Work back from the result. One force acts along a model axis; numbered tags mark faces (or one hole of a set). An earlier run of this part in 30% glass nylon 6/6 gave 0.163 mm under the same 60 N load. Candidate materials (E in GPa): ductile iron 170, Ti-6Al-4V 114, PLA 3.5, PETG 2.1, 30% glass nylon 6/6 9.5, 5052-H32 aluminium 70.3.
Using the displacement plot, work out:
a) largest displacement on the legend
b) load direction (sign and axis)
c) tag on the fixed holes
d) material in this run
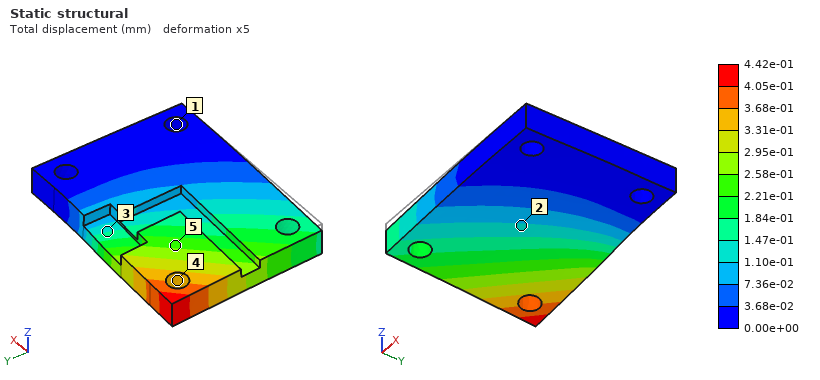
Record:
4.42e-01 mm
-Z
1
PLA
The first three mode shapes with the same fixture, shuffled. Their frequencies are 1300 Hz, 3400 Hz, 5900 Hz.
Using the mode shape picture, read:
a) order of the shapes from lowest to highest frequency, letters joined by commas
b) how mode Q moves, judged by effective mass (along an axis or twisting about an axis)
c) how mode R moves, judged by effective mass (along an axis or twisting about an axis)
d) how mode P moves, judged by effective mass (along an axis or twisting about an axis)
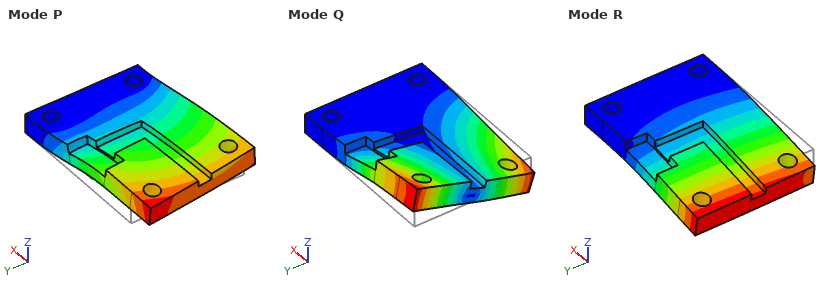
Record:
R, Q, P
twisting about X
along Z
along Y
